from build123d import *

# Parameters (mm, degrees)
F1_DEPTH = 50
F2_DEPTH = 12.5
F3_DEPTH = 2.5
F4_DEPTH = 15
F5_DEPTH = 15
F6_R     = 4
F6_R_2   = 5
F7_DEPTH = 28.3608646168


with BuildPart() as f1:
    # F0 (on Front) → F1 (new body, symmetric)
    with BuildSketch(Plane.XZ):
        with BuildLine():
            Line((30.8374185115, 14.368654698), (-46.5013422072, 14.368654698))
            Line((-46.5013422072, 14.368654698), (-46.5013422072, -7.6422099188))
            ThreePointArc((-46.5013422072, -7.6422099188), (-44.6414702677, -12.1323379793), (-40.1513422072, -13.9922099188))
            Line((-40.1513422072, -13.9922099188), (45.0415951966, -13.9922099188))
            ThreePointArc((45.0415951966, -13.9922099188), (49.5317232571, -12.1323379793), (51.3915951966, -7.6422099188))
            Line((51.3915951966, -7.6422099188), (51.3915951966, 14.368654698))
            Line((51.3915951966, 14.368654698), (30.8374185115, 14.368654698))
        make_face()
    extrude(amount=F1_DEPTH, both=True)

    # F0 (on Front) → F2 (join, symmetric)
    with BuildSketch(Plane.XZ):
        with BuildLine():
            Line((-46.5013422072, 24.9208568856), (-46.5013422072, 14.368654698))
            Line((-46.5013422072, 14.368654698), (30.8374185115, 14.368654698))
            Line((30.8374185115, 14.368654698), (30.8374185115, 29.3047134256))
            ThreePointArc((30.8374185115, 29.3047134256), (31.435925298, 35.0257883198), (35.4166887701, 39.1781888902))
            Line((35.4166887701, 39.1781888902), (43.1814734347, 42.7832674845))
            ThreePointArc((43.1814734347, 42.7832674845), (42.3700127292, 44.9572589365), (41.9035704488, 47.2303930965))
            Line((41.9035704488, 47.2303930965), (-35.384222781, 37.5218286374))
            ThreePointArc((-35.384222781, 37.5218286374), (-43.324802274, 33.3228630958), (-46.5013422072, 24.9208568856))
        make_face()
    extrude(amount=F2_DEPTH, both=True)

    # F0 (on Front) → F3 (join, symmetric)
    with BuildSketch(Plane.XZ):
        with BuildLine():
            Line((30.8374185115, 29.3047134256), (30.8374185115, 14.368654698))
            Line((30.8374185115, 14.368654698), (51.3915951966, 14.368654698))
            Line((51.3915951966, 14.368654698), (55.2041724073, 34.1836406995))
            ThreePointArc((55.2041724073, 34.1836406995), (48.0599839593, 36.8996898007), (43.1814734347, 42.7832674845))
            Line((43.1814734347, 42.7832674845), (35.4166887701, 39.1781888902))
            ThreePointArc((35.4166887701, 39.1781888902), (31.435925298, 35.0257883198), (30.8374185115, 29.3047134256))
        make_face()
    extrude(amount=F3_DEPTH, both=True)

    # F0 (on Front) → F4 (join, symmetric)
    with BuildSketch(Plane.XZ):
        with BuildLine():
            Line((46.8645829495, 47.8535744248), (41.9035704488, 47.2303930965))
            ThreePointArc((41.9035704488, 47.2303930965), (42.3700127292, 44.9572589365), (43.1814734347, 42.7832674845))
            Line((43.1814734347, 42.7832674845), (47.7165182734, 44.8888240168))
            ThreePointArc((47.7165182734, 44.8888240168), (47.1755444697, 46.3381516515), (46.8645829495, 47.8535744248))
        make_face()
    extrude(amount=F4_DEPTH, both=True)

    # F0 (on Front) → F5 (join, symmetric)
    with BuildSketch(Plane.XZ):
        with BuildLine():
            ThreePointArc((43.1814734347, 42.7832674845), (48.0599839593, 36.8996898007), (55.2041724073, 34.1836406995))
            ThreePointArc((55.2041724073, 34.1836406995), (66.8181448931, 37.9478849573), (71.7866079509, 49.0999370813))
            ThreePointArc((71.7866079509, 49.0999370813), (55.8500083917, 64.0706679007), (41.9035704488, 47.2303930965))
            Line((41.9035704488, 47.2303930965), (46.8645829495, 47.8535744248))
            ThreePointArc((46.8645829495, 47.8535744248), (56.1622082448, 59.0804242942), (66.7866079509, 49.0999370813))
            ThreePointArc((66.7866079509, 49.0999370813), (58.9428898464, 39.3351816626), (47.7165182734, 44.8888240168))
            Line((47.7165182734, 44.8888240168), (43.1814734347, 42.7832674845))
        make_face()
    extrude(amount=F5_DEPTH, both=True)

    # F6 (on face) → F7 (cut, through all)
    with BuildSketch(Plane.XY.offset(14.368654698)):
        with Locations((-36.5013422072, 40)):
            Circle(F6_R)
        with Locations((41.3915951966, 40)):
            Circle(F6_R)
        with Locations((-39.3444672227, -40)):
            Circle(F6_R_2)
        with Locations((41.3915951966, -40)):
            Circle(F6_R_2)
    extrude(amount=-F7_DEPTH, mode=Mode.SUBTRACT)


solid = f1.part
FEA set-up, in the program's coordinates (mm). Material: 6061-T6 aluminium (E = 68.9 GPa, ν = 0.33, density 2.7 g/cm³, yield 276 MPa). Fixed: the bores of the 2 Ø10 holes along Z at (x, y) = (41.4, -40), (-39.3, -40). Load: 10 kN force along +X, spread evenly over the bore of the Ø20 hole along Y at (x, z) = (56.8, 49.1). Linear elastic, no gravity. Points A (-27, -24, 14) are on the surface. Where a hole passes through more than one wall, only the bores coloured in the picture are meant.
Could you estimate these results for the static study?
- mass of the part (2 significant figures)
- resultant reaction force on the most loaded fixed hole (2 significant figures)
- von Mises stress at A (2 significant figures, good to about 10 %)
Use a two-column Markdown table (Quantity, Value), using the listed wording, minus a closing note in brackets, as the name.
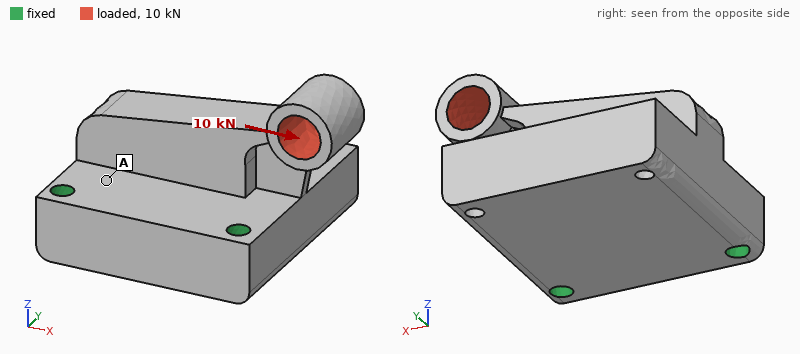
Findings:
| Quantity | Value |
|---|---|
| mass of the part | 910 g |
| resultant reaction force on the most loaded fixed hole | 9.1 kN |
| von Mises stress at A | 23 MPa |
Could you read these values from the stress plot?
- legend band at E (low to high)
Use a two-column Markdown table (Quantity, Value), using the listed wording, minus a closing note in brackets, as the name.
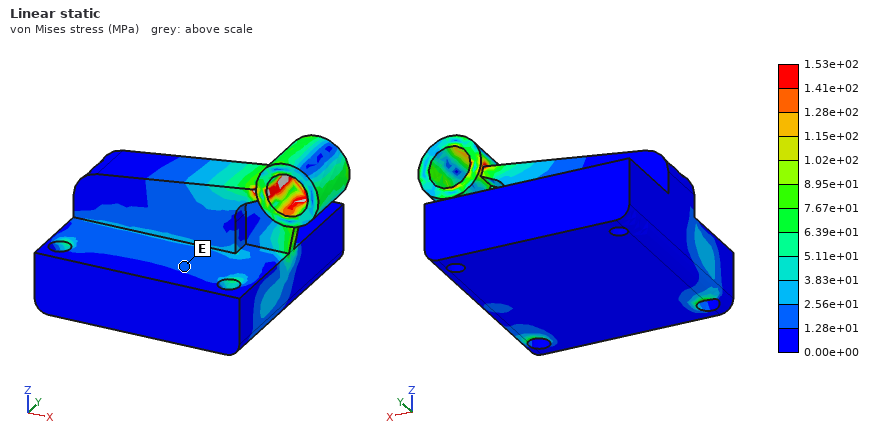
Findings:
| Quantity | Value |
|---|---|
| legend band at E | 1.28e+01 to 2.56e+01 MPa |
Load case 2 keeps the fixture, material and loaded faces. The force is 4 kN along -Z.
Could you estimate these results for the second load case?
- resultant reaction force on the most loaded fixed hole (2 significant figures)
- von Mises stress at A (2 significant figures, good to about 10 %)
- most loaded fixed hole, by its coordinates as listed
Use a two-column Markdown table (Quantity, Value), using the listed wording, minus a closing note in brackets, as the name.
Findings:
| Quantity | Value |
|---|---|
| resultant reaction force on the most loaded fixed hole | 4.7 kN |
| von Mises stress at A | 10 MPa |
| most loaded fixed hole, by its coordinates as listed | (41.4, -40) |
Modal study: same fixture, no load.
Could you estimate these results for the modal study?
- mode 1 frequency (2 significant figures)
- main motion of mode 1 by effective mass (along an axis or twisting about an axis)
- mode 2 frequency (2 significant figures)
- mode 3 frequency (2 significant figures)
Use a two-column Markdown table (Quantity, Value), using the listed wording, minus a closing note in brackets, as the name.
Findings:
| Quantity | Value |
|---|---|
| mode 1 frequency | 2000 Hz |
| main motion of mode 1 by effective mass | along Z |
| mode 2 frequency | 3700 Hz |
| mode 3 frequency | 4200 Hz |
